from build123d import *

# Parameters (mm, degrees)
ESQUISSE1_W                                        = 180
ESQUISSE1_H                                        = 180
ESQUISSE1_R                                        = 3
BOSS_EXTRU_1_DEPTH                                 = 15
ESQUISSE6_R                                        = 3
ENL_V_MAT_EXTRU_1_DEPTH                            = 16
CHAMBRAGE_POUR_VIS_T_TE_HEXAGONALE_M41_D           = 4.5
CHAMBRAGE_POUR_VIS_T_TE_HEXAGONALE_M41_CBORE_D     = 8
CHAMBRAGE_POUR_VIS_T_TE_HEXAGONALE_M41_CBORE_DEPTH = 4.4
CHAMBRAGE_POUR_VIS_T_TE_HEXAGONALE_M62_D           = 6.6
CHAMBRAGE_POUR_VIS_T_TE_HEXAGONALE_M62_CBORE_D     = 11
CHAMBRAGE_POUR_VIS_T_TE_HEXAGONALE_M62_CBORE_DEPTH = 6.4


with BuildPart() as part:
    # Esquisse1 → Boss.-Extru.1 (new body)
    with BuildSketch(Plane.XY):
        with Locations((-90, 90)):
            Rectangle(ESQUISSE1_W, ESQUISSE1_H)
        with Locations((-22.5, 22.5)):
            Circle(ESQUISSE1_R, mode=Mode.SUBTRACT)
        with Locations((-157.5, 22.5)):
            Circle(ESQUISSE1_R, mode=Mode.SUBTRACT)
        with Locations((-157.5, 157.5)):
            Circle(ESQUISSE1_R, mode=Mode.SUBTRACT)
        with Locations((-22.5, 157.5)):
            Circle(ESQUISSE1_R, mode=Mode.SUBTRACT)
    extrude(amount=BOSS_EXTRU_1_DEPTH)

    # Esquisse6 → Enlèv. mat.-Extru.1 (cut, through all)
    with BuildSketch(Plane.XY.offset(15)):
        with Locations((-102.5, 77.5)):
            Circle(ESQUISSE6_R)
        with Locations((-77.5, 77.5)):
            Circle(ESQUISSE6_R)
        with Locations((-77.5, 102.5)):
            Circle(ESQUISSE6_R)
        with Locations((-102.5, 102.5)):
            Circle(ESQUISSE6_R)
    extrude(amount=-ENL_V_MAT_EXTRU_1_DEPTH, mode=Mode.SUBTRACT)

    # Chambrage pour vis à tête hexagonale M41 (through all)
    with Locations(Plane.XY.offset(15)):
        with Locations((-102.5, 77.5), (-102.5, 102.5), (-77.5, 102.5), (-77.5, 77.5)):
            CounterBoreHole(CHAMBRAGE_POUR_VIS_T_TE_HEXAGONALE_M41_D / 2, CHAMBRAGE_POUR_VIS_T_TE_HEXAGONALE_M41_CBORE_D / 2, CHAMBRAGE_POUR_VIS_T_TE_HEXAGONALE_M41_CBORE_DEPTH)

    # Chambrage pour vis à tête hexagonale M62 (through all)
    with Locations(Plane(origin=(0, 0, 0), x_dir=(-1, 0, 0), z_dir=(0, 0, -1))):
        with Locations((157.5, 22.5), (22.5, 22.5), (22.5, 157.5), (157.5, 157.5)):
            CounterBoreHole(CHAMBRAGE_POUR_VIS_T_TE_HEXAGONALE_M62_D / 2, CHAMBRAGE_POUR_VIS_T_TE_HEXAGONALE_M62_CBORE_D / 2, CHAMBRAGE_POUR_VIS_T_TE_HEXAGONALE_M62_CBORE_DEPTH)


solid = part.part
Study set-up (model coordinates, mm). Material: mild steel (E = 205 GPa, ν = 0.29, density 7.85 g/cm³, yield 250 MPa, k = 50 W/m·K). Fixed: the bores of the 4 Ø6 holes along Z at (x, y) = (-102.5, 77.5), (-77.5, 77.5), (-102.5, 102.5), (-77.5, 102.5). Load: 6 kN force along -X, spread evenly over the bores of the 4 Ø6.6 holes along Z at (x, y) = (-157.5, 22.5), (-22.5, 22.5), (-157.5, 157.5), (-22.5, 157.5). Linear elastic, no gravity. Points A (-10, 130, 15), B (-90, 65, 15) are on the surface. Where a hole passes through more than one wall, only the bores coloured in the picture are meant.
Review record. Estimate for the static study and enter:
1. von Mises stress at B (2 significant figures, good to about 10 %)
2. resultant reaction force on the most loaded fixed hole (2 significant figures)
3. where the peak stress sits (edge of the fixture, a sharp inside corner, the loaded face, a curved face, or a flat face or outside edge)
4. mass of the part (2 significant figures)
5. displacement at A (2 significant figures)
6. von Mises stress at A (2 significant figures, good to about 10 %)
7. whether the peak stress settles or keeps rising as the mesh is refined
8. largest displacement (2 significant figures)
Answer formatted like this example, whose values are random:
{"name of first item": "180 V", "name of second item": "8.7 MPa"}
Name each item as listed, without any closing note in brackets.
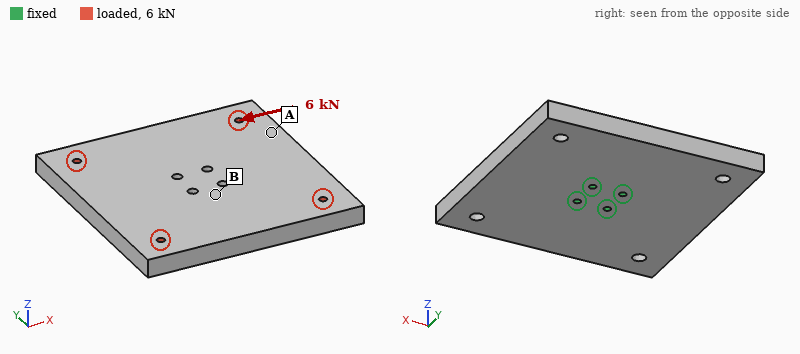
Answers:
{"von Mises stress at B": "5.2 MPa", "resultant reaction force on the most loaded fixed hole": "1.6 kN", "where the peak stress sits": "edge of the fixture", "mass of the part": "3.8 kg", "displacement at A": "4.5 µm", "von Mises stress at A": "2.0 MPa", "whether the peak stress settles or keeps rising as the mesh is refined": "keeps rising", "largest displacement": "6.5 µm"}
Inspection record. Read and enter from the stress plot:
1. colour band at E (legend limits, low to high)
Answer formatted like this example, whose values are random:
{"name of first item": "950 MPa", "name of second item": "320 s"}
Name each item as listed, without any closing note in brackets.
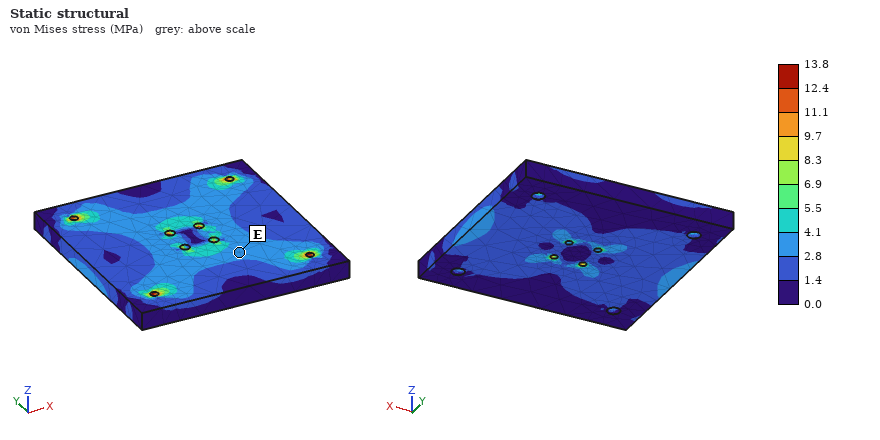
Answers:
{"colour band at E": "2.8 to 4.1 MPa"}
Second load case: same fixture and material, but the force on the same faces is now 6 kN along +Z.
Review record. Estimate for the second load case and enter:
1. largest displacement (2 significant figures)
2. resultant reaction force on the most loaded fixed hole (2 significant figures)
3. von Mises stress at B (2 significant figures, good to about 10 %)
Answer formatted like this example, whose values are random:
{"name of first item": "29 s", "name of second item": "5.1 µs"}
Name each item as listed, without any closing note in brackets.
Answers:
{"largest displacement": "62 µm", "resultant reaction force on the most loaded fixed hole": "2.2 kN", "von Mises stress at B": "23 MPa"}
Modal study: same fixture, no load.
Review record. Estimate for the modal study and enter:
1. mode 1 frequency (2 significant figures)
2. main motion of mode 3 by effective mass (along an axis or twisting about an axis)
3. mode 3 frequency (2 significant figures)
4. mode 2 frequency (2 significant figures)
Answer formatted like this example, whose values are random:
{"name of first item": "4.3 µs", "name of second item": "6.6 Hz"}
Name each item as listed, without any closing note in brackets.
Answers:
{"mode 1 frequency": "1200 Hz", "main motion of mode 3 by effective mass": "along Z", "mode 3 frequency": "1500 Hz", "mode 2 frequency": "1200 Hz"}
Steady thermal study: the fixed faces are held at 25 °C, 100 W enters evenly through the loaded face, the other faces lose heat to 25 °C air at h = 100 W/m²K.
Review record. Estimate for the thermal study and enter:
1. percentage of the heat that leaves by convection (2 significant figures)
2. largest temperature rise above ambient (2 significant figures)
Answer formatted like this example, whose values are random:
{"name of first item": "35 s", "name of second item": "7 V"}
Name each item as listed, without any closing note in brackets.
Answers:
{"percentage of the heat that leaves by convection": "76 %", "largest temperature rise above ambient": "30 K"}
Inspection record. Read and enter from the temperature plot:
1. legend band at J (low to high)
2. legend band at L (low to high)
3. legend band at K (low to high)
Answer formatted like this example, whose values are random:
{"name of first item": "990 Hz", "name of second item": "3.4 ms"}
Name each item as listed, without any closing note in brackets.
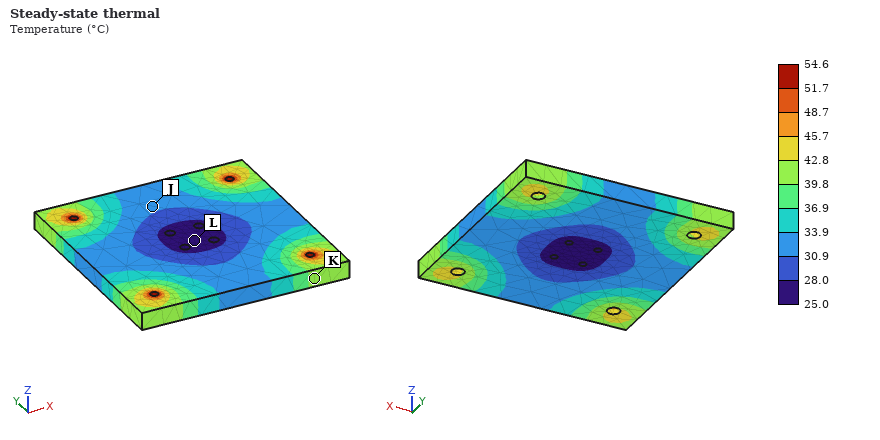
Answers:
{"legend band at J": "30.9 to 33.9 °C", "legend band at L": "25.0 to 28.0 °C", "legend band at K": "39.8 to 42.8 °C"}
